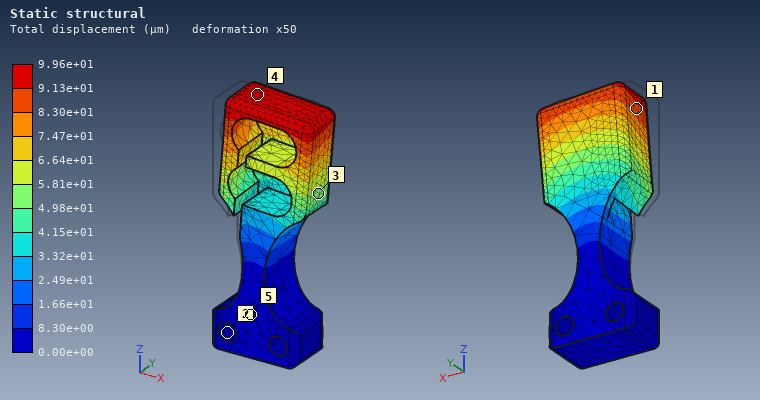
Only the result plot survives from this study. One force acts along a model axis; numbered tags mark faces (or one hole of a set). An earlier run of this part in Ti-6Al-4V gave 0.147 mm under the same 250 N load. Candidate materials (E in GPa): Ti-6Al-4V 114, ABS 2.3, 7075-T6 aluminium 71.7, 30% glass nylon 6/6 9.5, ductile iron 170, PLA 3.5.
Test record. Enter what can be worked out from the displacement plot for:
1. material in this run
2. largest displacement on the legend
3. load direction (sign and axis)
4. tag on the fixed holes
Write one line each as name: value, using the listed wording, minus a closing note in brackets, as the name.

material in this run: ductile iron
largest displacement on the legend: 9.96e+01 µm
load direction: +X
tag on the fixed holes: 2
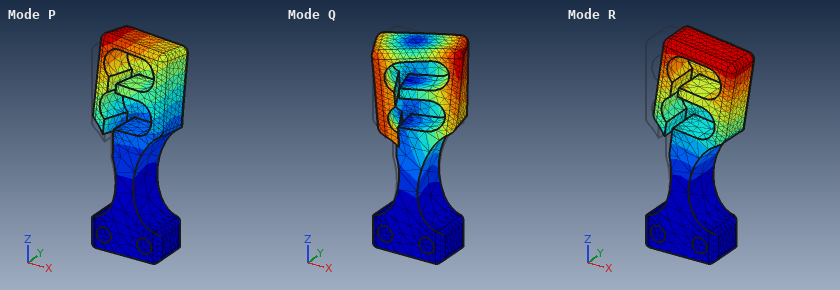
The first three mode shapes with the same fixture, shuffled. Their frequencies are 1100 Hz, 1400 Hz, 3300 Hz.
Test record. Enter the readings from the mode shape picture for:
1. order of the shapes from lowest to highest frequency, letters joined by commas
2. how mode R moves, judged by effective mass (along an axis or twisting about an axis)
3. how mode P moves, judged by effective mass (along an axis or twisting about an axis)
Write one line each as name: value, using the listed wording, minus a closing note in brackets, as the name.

order of the shapes from lowest to highest frequency, letters joined by commas: R, P, Q
how mode R moves, judged by effective mass: along X
how mode P moves, judged by effective mass: along Y
